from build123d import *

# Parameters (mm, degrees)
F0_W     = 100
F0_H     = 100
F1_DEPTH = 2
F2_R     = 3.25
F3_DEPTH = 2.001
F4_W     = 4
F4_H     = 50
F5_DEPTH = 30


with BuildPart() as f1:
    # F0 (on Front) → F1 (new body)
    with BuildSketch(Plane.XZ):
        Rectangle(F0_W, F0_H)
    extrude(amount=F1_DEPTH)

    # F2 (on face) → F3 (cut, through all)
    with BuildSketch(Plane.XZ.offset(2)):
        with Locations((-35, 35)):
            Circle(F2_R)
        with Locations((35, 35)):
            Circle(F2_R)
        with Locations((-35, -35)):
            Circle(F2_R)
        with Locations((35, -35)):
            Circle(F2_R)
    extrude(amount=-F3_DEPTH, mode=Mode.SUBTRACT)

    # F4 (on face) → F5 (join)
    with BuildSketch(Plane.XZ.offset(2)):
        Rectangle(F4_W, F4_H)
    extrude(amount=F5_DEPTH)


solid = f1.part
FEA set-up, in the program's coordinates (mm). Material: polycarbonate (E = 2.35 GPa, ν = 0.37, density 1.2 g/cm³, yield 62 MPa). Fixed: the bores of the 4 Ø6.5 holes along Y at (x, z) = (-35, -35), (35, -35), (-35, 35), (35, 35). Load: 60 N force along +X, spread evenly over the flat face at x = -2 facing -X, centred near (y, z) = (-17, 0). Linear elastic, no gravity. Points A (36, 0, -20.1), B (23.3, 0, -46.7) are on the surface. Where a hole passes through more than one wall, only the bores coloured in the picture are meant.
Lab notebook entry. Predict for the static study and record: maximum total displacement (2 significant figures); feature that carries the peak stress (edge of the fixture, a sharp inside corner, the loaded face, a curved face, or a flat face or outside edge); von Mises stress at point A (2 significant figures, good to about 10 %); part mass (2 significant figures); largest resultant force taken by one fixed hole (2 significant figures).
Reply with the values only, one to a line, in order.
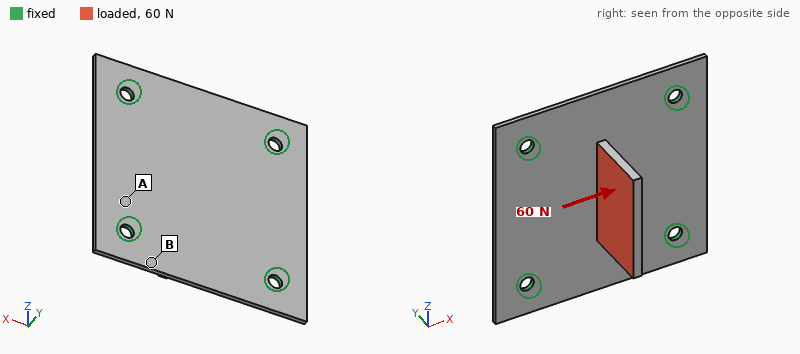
1.5 mm
a flat face or outside edge
1.5 MPa
31 g
19 N
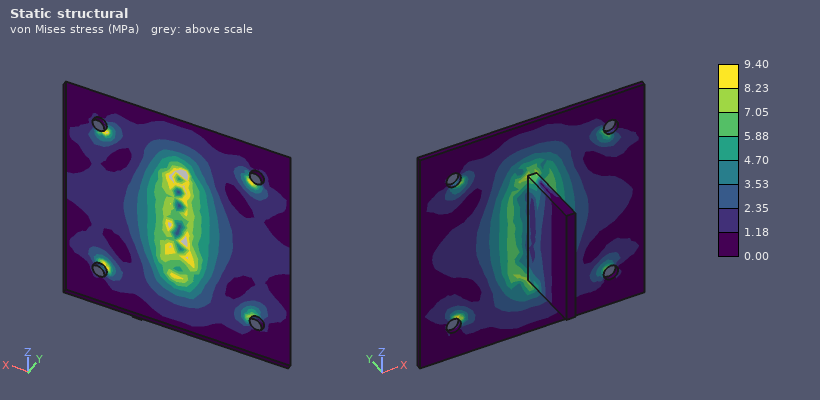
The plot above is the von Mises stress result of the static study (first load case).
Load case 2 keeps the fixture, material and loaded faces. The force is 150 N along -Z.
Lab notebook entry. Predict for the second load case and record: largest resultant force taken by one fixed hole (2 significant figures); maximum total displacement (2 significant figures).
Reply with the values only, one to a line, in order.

45 N
1.4 mm
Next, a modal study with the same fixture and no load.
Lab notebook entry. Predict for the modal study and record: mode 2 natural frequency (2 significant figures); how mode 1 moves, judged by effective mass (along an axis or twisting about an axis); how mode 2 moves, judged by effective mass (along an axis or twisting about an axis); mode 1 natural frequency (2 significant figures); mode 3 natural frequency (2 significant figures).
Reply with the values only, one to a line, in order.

440 Hz
along Y
along X
360 Hz
500 Hz
